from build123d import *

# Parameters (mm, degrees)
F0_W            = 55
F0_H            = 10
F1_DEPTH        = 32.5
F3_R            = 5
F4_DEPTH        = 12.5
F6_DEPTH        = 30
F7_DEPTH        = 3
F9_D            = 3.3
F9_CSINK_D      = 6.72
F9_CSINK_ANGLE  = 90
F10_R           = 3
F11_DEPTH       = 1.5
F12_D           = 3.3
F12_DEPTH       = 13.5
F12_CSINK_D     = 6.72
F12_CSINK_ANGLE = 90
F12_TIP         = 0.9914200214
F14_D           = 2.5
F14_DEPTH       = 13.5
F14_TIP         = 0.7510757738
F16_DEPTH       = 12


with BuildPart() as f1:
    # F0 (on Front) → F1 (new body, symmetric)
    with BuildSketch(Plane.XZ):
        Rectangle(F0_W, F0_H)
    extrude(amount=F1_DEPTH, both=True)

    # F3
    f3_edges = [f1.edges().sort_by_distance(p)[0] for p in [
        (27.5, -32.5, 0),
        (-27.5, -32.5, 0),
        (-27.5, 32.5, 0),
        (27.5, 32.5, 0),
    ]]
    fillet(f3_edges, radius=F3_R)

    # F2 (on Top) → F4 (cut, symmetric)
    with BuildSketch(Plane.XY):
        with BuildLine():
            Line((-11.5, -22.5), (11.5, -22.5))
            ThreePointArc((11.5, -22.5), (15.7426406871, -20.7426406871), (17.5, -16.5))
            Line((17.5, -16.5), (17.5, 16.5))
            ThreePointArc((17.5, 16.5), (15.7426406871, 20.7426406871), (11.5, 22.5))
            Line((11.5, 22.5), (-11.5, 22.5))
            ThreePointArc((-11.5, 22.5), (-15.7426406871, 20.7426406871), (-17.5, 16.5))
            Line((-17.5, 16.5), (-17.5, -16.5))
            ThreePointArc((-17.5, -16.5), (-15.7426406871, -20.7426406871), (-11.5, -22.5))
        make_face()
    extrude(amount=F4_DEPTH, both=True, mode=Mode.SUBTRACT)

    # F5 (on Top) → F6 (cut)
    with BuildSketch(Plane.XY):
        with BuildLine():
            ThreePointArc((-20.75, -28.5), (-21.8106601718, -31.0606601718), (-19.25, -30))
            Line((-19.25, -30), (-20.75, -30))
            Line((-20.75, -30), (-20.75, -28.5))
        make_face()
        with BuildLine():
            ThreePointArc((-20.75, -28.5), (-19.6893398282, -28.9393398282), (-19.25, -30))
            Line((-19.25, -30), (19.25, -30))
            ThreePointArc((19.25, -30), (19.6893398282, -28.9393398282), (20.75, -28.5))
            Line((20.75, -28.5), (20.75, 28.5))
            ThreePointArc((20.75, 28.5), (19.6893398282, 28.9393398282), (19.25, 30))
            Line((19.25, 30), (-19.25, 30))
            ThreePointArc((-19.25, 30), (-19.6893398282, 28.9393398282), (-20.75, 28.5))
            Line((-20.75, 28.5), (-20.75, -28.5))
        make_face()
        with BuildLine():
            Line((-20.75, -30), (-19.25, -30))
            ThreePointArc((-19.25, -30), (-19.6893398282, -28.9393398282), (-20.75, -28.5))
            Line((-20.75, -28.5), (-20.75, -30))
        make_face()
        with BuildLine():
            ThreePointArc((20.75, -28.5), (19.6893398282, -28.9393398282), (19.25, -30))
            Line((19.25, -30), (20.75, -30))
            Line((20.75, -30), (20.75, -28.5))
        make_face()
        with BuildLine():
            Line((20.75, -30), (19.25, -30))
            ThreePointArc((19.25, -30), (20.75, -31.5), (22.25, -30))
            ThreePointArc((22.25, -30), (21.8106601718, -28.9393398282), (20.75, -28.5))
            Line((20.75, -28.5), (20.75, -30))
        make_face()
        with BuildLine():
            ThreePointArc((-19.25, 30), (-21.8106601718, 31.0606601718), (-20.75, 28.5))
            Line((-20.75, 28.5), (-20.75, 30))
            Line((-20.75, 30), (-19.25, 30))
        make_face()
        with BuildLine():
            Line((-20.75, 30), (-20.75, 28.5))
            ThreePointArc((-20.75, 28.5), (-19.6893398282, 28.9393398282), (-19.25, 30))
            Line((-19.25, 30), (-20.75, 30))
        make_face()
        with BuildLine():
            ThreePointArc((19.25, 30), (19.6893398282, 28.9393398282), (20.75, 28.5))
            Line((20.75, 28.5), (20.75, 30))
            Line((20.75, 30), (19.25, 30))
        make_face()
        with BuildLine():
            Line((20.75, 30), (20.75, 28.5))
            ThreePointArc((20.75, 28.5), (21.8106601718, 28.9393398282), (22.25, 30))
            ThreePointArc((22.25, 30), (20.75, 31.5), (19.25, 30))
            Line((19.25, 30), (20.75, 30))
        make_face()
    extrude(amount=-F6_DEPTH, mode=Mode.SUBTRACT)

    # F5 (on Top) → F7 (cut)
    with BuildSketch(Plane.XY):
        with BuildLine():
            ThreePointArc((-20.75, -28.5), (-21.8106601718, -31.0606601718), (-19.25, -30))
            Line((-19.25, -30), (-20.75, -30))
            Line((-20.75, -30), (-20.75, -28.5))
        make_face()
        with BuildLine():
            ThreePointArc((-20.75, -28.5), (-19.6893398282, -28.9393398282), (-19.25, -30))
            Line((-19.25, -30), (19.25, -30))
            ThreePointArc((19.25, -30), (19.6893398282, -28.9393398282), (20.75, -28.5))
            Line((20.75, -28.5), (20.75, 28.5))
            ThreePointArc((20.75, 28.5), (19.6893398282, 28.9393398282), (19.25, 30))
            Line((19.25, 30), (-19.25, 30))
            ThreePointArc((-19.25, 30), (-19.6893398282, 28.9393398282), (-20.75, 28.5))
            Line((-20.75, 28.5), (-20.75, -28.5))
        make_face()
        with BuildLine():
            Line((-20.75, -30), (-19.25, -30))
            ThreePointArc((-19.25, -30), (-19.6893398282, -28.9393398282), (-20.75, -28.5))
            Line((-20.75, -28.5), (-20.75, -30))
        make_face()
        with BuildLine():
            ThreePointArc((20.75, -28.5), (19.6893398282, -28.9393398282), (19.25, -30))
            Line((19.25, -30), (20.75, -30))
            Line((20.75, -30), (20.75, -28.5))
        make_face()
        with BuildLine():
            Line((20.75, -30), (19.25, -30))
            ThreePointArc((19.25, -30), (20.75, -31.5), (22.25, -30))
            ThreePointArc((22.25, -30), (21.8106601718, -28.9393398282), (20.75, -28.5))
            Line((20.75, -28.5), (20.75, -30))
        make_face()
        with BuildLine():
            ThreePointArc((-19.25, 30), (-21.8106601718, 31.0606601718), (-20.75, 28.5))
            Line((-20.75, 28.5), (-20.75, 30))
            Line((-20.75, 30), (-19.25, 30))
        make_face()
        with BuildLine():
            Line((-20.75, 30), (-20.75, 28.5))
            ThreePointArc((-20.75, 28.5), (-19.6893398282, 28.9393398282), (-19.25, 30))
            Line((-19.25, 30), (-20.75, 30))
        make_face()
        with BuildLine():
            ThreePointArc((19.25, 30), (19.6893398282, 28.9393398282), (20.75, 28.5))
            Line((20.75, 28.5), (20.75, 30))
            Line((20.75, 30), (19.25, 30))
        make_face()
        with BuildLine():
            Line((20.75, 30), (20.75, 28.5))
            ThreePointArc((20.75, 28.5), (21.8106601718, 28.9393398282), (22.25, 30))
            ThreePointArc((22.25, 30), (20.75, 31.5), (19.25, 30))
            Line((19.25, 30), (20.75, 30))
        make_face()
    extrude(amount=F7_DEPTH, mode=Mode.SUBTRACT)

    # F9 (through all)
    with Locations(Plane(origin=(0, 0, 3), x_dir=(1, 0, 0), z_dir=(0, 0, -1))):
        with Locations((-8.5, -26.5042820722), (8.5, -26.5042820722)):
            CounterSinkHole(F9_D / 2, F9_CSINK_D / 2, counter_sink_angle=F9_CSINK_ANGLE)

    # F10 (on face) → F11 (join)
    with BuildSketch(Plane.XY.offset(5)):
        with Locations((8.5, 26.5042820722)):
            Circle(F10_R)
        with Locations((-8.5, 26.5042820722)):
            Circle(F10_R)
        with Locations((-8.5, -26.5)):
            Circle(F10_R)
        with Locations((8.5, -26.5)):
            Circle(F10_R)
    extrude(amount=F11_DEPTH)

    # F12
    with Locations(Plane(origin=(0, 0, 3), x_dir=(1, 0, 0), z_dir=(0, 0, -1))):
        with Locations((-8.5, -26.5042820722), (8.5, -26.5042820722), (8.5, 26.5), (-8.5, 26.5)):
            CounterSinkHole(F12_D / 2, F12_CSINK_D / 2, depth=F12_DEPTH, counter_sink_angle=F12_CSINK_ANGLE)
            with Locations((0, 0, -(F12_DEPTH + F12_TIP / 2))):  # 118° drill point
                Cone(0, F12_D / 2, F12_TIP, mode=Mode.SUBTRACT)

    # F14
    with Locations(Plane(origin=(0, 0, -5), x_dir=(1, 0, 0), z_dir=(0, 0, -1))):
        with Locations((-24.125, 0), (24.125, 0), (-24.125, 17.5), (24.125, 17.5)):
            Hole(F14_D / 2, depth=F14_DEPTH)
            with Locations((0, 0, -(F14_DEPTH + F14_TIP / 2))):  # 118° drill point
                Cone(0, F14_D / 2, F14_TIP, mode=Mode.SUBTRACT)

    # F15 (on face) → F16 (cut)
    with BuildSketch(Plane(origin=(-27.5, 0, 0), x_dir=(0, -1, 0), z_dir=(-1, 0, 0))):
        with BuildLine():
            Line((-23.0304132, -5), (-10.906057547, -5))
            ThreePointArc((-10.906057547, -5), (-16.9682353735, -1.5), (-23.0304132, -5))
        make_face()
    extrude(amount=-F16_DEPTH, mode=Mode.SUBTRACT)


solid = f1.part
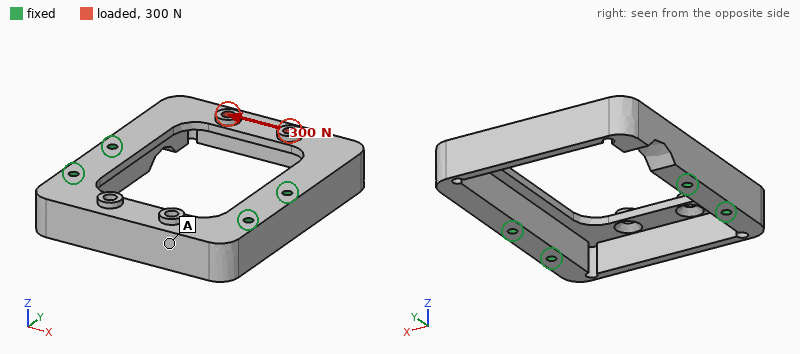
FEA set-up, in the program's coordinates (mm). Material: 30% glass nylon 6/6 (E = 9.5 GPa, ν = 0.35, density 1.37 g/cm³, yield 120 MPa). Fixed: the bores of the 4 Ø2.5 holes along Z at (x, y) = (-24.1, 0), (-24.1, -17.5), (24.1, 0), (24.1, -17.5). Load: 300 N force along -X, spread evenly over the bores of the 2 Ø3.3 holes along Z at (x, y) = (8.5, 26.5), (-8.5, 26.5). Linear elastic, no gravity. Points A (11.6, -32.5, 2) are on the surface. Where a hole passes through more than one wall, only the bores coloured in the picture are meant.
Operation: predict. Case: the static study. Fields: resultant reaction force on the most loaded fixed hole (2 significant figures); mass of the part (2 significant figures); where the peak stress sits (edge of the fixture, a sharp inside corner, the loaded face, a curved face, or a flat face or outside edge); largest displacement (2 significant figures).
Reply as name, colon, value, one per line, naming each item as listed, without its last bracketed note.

resultant reaction force on the most loaded fixed hole: 240 N
mass of the part: 16 g
where the peak stress sits: a curved face
largest displacement: 0.20 mm
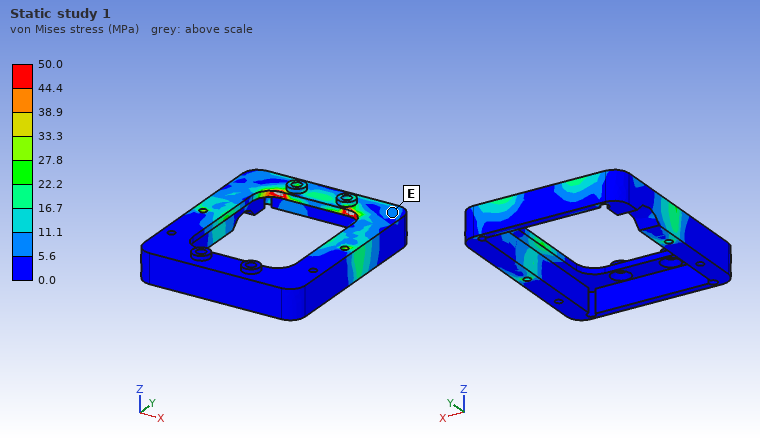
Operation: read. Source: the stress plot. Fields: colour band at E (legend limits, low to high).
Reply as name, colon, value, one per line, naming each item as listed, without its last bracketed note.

colour band at E: 5.6 to 11.1 MPa
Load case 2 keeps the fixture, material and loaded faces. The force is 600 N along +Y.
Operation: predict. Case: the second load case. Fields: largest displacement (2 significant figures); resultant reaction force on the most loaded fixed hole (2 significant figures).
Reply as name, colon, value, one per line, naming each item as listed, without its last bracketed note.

largest displacement: 0.26 mm
resultant reaction force on the most loaded fixed hole: 330 N
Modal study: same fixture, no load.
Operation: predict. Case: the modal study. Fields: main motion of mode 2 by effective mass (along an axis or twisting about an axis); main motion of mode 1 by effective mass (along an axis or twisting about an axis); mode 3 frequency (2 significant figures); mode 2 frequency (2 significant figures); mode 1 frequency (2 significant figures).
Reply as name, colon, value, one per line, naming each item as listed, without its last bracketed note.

main motion of mode 2 by effective mass: along X
main motion of mode 1 by effective mass: along Z
mode 3 frequency: 4000 Hz
mode 2 frequency: 2900 Hz
mode 1 frequency: 2400 Hz
